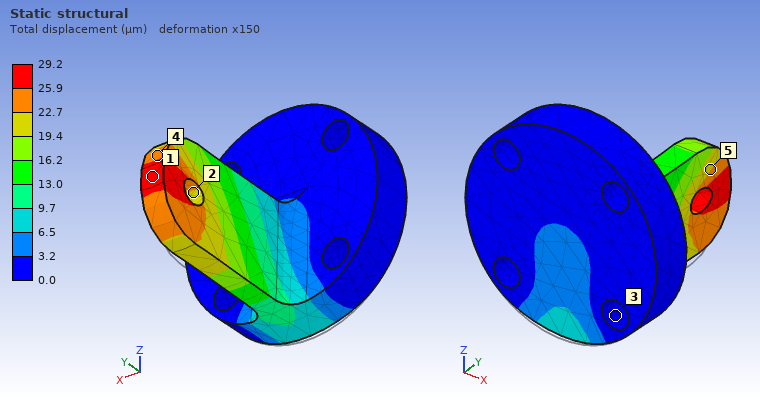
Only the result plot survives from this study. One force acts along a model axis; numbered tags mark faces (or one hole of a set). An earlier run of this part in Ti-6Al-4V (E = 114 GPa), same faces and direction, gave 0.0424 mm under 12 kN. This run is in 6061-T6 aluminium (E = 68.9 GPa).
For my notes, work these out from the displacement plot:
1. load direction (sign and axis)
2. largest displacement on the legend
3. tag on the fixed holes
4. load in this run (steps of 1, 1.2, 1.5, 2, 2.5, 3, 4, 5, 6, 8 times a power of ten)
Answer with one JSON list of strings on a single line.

["+Y", "29.2 µm", "3", "5 kN"]
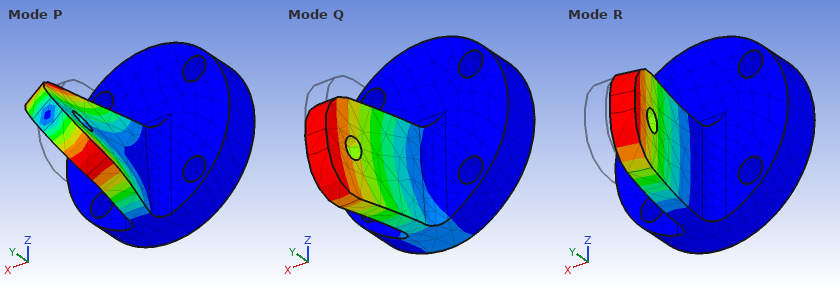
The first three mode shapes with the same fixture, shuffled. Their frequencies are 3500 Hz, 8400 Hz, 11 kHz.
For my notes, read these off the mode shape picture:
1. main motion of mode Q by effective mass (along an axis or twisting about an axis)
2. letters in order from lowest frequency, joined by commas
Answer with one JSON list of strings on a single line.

["along Z", "R, Q, P"]
